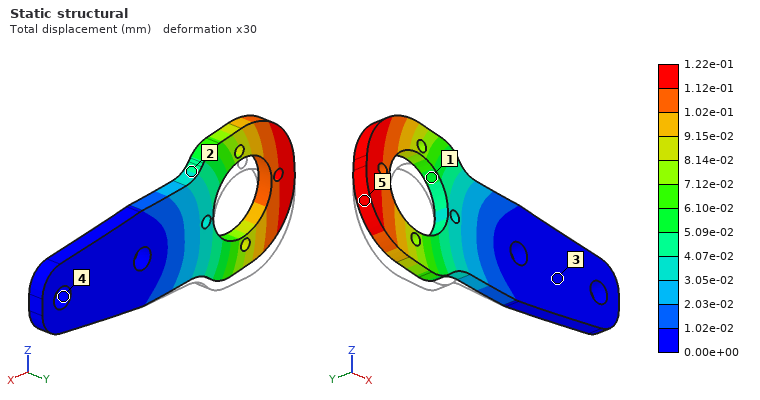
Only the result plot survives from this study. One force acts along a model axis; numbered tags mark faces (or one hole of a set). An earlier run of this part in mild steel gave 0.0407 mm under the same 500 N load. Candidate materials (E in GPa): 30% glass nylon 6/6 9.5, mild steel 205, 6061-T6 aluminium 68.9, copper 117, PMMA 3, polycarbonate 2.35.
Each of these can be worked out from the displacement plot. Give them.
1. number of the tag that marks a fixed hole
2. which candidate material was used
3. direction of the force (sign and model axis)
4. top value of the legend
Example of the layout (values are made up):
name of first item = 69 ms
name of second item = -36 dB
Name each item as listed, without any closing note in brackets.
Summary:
number of the tag that marks a fixed hole = 4
which candidate material was used = 6061-T6 aluminium
direction of the force = +Z
top value of the legend = 1.22e-01 mm
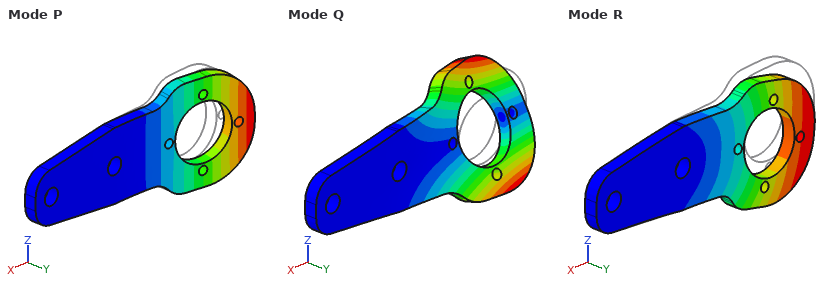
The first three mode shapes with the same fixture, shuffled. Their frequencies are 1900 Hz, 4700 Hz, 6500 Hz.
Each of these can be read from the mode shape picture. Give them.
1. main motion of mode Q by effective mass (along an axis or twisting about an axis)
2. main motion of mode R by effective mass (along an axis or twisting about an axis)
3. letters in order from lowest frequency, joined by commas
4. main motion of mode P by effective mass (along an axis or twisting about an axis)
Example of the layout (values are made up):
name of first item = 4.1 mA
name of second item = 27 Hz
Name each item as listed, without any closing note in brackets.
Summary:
main motion of mode Q by effective mass = twisting about X
main motion of mode R by effective mass = along Z
letters in order from lowest frequency, joined by commas = P, Q, R
main motion of mode P by effective mass = along Y
